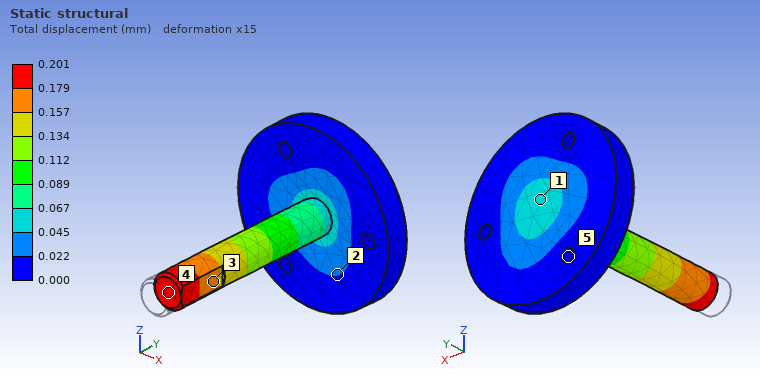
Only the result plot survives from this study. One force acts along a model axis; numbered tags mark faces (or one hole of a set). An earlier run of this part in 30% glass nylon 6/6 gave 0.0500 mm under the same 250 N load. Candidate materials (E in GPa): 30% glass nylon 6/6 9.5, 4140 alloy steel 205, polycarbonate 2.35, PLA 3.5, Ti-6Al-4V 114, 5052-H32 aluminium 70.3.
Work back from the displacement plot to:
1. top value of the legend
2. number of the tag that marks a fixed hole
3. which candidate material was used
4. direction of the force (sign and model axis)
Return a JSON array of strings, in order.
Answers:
["0.201 mm", "5", "polycarbonate", "+Y"]
